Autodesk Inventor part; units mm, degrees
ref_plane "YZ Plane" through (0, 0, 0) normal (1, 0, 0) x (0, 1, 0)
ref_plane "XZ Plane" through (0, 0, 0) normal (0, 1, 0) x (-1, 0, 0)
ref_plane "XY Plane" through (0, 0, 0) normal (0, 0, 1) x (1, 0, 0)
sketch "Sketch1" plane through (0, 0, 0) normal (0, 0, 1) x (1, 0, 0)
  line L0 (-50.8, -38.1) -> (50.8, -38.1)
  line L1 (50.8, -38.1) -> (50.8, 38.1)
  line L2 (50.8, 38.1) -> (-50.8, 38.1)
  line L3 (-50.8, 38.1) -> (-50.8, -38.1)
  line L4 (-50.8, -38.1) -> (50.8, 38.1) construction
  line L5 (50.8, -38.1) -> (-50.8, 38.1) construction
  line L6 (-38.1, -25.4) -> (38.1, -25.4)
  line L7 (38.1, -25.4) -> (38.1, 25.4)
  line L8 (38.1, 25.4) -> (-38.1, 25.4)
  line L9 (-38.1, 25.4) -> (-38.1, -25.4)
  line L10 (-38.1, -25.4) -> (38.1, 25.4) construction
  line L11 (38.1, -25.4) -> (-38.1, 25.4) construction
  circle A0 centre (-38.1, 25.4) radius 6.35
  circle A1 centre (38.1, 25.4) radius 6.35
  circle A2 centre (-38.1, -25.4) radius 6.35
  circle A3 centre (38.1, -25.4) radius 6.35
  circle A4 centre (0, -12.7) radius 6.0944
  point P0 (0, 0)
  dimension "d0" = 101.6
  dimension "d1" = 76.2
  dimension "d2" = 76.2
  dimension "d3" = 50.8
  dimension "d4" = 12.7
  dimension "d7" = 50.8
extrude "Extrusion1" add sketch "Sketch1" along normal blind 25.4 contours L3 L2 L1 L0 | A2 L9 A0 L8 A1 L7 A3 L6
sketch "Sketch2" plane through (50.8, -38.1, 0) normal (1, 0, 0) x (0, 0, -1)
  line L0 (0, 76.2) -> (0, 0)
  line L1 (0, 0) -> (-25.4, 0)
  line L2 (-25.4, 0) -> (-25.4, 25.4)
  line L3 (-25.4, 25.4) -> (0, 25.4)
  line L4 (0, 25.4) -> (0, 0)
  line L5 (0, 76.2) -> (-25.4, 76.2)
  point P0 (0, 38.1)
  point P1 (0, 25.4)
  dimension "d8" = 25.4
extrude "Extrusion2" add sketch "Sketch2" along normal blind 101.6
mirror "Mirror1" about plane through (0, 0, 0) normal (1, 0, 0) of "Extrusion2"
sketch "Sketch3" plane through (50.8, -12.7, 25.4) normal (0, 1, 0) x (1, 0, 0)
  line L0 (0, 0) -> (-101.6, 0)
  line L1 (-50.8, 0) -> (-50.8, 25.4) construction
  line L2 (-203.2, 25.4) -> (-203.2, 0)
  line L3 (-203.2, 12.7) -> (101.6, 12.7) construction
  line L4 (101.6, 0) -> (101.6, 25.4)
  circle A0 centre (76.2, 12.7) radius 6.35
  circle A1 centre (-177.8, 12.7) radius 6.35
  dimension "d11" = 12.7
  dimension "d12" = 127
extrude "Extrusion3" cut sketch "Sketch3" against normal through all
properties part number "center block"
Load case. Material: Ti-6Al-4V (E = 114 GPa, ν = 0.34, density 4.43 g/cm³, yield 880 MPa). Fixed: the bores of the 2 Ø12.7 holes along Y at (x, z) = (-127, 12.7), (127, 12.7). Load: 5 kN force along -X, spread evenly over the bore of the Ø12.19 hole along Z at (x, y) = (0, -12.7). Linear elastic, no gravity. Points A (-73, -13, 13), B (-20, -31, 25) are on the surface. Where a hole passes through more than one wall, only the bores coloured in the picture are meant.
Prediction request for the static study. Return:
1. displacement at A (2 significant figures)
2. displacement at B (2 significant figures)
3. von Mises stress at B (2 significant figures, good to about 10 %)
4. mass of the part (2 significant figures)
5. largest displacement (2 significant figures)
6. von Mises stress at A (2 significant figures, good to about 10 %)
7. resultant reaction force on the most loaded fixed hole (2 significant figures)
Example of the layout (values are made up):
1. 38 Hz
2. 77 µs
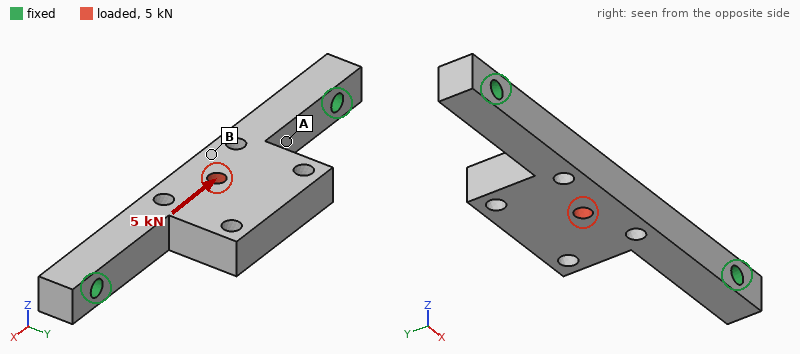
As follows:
1. 2.6 µm
2. 3.5 µm
3. 2.0 MPa
4. 1.4 kg
5. 7.4 µm
6. 6.3 MPa
7. 2.5 kN
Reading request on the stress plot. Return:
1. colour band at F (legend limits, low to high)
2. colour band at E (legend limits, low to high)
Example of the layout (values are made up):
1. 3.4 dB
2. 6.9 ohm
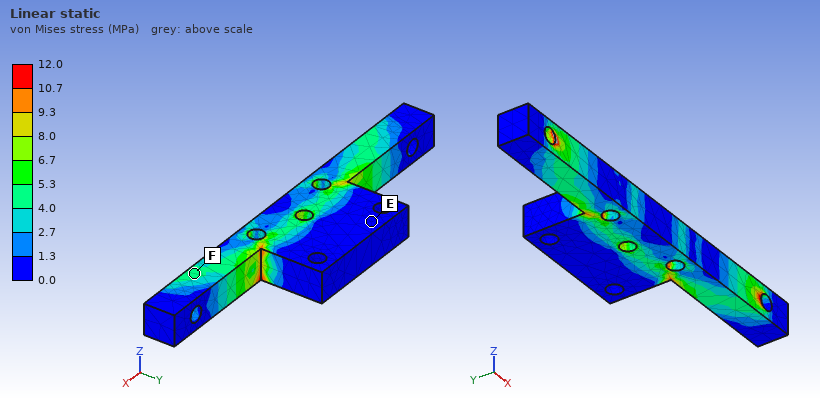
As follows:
1. 4.0 to 5.3 MPa
2. 0.0 to 1.3 MPa
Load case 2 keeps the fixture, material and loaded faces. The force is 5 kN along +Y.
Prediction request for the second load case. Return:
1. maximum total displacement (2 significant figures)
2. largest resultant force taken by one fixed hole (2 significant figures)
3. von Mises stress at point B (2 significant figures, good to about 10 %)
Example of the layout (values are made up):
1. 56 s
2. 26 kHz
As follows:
1. 48 µm
2. 2.9 kN
3. 6.2 MPa
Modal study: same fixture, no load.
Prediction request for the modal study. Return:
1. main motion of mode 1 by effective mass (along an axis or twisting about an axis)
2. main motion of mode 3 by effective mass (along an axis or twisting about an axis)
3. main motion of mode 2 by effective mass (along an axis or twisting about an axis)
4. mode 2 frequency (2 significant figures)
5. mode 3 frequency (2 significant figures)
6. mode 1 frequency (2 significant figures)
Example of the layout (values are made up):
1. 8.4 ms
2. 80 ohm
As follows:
1. along Z
2. along Z
3. along Y
4. 1800 Hz
5. 2300 Hz
6. 970 Hz
